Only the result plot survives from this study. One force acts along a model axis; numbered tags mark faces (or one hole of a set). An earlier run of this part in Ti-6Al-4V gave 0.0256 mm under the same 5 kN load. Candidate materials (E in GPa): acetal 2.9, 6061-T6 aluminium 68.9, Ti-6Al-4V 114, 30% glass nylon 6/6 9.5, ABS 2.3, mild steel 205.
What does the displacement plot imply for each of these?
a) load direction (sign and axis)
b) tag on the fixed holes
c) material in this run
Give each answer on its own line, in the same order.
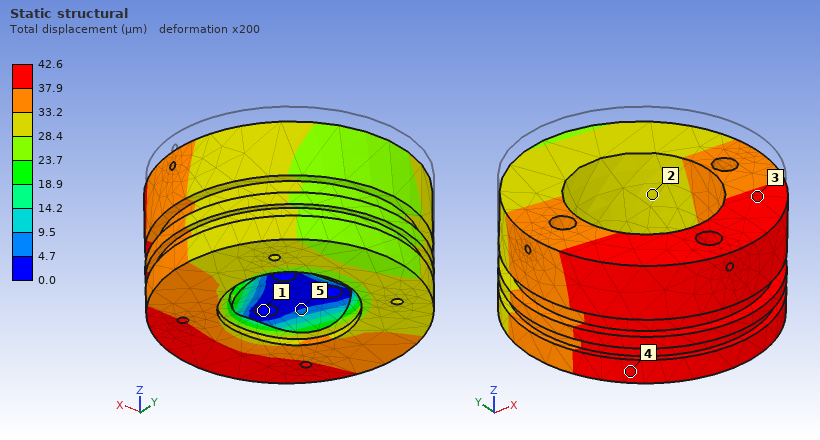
-Z
1
6061-T6 aluminium
